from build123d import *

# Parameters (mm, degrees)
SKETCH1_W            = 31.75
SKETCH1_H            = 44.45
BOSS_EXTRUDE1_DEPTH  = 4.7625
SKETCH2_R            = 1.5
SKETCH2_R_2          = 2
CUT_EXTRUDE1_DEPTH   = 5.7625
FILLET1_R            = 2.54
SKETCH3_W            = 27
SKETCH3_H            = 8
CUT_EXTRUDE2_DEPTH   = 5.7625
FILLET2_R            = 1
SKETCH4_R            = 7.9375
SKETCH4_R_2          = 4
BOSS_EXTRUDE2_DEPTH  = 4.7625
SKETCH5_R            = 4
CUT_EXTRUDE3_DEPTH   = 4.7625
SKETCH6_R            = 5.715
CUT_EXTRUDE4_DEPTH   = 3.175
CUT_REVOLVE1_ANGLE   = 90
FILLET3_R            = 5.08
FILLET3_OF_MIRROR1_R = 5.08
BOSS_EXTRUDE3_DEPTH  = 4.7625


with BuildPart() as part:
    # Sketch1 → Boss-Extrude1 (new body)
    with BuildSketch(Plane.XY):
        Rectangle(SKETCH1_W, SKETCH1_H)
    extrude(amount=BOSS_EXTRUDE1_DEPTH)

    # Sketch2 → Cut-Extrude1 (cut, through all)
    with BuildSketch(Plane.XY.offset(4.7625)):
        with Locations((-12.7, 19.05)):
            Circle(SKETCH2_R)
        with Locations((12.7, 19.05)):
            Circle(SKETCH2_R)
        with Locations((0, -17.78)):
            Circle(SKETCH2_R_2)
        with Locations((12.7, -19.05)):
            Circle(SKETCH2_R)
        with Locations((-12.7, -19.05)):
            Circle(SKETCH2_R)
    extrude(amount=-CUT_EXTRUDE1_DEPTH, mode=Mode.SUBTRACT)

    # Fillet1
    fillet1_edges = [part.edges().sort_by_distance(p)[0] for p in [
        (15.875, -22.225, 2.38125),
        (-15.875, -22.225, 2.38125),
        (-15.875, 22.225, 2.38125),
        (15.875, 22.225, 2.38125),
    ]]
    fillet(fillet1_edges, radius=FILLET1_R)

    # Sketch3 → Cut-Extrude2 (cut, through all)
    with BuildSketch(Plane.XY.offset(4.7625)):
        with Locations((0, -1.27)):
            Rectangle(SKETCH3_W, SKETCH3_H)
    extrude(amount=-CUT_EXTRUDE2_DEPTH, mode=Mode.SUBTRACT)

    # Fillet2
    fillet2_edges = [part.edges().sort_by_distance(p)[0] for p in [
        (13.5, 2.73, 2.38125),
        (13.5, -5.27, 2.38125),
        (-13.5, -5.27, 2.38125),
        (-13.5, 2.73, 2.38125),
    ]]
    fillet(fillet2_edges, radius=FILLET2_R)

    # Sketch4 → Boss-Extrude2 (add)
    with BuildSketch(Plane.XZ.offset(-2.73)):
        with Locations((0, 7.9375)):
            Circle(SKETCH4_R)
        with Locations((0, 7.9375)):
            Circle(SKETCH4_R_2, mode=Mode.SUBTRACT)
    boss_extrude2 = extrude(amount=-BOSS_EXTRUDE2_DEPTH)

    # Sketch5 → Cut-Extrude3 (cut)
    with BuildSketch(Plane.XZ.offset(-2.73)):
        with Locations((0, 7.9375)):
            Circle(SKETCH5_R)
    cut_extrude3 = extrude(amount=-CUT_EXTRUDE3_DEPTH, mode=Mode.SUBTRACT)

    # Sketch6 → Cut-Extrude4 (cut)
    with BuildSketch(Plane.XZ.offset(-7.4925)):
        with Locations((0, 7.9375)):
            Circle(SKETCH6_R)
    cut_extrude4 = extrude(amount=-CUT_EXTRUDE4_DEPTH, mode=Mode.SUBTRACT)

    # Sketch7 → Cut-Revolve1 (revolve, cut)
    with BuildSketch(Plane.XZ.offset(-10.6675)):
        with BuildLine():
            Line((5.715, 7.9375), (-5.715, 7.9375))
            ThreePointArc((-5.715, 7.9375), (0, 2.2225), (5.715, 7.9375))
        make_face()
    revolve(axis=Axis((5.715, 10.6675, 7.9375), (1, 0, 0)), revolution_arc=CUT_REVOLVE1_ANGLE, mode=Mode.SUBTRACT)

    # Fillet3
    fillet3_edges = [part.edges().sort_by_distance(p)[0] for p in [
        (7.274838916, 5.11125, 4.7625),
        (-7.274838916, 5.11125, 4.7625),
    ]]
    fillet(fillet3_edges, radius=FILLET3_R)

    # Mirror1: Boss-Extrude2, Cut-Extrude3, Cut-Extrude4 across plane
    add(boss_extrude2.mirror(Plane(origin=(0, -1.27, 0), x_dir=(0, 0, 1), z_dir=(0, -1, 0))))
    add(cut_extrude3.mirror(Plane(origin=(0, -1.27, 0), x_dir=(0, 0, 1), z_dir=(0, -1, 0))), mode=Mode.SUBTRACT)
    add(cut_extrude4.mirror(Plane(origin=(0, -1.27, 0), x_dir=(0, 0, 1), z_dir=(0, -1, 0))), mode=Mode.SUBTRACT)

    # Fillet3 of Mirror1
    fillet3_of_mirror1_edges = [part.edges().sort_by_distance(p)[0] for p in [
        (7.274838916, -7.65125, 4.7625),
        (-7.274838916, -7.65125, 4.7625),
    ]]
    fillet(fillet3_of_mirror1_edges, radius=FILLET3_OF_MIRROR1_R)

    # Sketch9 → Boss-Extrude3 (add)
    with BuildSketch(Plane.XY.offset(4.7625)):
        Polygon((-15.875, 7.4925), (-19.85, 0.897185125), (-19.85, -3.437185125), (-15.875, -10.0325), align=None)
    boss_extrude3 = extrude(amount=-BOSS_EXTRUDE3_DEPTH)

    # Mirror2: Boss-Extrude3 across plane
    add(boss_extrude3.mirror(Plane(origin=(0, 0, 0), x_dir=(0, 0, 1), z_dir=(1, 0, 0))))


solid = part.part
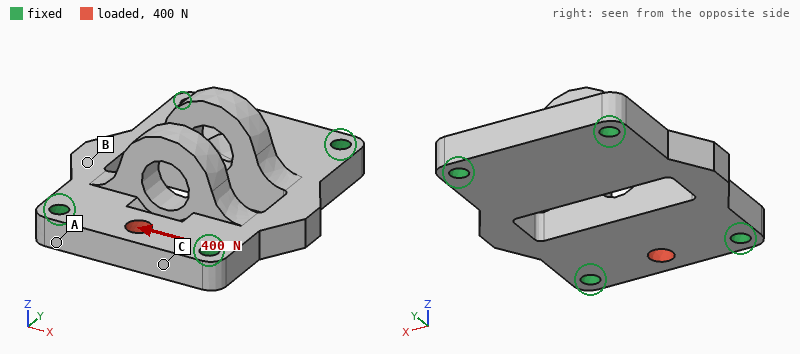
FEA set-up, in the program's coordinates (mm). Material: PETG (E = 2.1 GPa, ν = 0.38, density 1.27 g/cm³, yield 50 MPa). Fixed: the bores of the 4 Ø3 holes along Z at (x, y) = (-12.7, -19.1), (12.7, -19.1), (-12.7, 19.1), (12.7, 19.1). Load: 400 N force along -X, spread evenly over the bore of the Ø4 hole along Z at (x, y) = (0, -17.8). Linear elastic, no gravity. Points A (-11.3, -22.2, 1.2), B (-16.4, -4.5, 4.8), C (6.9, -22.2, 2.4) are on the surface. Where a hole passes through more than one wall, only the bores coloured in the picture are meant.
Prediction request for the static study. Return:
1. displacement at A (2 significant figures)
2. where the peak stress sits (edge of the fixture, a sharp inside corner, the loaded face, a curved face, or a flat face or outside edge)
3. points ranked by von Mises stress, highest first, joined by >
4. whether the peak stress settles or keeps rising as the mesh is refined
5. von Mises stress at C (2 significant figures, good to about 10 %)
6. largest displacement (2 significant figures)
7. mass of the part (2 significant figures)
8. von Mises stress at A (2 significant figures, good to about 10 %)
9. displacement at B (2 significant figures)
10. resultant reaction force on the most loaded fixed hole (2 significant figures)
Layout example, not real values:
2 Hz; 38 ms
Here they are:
5.6 µm; edge of the fixture; C > A > B; keeps rising; 4.8 MPa; 31 µm; 8.6 g; 2.8 MPa; 14 µm; 200 N
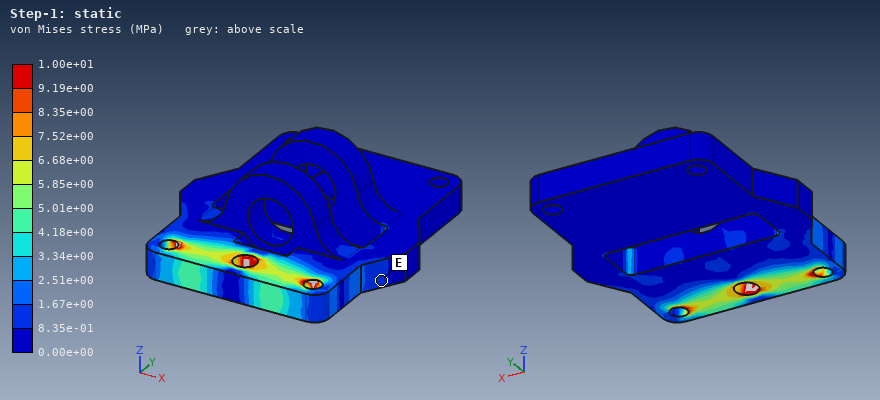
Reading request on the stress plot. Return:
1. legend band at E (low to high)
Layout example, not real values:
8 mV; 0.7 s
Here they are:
8.35e-01 to 1.67e+00 MPa
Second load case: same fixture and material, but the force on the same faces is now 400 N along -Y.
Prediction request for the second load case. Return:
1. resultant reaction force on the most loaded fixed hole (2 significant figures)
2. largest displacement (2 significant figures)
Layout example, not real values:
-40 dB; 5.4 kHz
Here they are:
210 N; 93 µm
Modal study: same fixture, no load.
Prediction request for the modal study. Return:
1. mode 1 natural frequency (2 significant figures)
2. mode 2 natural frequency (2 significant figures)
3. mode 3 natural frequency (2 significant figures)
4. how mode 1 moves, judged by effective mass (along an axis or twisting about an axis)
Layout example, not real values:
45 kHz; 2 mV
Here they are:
2500 Hz; 3800 Hz; 3800 Hz; along Z
